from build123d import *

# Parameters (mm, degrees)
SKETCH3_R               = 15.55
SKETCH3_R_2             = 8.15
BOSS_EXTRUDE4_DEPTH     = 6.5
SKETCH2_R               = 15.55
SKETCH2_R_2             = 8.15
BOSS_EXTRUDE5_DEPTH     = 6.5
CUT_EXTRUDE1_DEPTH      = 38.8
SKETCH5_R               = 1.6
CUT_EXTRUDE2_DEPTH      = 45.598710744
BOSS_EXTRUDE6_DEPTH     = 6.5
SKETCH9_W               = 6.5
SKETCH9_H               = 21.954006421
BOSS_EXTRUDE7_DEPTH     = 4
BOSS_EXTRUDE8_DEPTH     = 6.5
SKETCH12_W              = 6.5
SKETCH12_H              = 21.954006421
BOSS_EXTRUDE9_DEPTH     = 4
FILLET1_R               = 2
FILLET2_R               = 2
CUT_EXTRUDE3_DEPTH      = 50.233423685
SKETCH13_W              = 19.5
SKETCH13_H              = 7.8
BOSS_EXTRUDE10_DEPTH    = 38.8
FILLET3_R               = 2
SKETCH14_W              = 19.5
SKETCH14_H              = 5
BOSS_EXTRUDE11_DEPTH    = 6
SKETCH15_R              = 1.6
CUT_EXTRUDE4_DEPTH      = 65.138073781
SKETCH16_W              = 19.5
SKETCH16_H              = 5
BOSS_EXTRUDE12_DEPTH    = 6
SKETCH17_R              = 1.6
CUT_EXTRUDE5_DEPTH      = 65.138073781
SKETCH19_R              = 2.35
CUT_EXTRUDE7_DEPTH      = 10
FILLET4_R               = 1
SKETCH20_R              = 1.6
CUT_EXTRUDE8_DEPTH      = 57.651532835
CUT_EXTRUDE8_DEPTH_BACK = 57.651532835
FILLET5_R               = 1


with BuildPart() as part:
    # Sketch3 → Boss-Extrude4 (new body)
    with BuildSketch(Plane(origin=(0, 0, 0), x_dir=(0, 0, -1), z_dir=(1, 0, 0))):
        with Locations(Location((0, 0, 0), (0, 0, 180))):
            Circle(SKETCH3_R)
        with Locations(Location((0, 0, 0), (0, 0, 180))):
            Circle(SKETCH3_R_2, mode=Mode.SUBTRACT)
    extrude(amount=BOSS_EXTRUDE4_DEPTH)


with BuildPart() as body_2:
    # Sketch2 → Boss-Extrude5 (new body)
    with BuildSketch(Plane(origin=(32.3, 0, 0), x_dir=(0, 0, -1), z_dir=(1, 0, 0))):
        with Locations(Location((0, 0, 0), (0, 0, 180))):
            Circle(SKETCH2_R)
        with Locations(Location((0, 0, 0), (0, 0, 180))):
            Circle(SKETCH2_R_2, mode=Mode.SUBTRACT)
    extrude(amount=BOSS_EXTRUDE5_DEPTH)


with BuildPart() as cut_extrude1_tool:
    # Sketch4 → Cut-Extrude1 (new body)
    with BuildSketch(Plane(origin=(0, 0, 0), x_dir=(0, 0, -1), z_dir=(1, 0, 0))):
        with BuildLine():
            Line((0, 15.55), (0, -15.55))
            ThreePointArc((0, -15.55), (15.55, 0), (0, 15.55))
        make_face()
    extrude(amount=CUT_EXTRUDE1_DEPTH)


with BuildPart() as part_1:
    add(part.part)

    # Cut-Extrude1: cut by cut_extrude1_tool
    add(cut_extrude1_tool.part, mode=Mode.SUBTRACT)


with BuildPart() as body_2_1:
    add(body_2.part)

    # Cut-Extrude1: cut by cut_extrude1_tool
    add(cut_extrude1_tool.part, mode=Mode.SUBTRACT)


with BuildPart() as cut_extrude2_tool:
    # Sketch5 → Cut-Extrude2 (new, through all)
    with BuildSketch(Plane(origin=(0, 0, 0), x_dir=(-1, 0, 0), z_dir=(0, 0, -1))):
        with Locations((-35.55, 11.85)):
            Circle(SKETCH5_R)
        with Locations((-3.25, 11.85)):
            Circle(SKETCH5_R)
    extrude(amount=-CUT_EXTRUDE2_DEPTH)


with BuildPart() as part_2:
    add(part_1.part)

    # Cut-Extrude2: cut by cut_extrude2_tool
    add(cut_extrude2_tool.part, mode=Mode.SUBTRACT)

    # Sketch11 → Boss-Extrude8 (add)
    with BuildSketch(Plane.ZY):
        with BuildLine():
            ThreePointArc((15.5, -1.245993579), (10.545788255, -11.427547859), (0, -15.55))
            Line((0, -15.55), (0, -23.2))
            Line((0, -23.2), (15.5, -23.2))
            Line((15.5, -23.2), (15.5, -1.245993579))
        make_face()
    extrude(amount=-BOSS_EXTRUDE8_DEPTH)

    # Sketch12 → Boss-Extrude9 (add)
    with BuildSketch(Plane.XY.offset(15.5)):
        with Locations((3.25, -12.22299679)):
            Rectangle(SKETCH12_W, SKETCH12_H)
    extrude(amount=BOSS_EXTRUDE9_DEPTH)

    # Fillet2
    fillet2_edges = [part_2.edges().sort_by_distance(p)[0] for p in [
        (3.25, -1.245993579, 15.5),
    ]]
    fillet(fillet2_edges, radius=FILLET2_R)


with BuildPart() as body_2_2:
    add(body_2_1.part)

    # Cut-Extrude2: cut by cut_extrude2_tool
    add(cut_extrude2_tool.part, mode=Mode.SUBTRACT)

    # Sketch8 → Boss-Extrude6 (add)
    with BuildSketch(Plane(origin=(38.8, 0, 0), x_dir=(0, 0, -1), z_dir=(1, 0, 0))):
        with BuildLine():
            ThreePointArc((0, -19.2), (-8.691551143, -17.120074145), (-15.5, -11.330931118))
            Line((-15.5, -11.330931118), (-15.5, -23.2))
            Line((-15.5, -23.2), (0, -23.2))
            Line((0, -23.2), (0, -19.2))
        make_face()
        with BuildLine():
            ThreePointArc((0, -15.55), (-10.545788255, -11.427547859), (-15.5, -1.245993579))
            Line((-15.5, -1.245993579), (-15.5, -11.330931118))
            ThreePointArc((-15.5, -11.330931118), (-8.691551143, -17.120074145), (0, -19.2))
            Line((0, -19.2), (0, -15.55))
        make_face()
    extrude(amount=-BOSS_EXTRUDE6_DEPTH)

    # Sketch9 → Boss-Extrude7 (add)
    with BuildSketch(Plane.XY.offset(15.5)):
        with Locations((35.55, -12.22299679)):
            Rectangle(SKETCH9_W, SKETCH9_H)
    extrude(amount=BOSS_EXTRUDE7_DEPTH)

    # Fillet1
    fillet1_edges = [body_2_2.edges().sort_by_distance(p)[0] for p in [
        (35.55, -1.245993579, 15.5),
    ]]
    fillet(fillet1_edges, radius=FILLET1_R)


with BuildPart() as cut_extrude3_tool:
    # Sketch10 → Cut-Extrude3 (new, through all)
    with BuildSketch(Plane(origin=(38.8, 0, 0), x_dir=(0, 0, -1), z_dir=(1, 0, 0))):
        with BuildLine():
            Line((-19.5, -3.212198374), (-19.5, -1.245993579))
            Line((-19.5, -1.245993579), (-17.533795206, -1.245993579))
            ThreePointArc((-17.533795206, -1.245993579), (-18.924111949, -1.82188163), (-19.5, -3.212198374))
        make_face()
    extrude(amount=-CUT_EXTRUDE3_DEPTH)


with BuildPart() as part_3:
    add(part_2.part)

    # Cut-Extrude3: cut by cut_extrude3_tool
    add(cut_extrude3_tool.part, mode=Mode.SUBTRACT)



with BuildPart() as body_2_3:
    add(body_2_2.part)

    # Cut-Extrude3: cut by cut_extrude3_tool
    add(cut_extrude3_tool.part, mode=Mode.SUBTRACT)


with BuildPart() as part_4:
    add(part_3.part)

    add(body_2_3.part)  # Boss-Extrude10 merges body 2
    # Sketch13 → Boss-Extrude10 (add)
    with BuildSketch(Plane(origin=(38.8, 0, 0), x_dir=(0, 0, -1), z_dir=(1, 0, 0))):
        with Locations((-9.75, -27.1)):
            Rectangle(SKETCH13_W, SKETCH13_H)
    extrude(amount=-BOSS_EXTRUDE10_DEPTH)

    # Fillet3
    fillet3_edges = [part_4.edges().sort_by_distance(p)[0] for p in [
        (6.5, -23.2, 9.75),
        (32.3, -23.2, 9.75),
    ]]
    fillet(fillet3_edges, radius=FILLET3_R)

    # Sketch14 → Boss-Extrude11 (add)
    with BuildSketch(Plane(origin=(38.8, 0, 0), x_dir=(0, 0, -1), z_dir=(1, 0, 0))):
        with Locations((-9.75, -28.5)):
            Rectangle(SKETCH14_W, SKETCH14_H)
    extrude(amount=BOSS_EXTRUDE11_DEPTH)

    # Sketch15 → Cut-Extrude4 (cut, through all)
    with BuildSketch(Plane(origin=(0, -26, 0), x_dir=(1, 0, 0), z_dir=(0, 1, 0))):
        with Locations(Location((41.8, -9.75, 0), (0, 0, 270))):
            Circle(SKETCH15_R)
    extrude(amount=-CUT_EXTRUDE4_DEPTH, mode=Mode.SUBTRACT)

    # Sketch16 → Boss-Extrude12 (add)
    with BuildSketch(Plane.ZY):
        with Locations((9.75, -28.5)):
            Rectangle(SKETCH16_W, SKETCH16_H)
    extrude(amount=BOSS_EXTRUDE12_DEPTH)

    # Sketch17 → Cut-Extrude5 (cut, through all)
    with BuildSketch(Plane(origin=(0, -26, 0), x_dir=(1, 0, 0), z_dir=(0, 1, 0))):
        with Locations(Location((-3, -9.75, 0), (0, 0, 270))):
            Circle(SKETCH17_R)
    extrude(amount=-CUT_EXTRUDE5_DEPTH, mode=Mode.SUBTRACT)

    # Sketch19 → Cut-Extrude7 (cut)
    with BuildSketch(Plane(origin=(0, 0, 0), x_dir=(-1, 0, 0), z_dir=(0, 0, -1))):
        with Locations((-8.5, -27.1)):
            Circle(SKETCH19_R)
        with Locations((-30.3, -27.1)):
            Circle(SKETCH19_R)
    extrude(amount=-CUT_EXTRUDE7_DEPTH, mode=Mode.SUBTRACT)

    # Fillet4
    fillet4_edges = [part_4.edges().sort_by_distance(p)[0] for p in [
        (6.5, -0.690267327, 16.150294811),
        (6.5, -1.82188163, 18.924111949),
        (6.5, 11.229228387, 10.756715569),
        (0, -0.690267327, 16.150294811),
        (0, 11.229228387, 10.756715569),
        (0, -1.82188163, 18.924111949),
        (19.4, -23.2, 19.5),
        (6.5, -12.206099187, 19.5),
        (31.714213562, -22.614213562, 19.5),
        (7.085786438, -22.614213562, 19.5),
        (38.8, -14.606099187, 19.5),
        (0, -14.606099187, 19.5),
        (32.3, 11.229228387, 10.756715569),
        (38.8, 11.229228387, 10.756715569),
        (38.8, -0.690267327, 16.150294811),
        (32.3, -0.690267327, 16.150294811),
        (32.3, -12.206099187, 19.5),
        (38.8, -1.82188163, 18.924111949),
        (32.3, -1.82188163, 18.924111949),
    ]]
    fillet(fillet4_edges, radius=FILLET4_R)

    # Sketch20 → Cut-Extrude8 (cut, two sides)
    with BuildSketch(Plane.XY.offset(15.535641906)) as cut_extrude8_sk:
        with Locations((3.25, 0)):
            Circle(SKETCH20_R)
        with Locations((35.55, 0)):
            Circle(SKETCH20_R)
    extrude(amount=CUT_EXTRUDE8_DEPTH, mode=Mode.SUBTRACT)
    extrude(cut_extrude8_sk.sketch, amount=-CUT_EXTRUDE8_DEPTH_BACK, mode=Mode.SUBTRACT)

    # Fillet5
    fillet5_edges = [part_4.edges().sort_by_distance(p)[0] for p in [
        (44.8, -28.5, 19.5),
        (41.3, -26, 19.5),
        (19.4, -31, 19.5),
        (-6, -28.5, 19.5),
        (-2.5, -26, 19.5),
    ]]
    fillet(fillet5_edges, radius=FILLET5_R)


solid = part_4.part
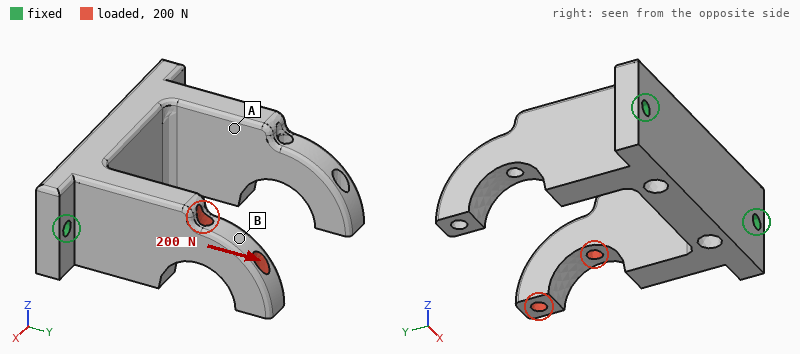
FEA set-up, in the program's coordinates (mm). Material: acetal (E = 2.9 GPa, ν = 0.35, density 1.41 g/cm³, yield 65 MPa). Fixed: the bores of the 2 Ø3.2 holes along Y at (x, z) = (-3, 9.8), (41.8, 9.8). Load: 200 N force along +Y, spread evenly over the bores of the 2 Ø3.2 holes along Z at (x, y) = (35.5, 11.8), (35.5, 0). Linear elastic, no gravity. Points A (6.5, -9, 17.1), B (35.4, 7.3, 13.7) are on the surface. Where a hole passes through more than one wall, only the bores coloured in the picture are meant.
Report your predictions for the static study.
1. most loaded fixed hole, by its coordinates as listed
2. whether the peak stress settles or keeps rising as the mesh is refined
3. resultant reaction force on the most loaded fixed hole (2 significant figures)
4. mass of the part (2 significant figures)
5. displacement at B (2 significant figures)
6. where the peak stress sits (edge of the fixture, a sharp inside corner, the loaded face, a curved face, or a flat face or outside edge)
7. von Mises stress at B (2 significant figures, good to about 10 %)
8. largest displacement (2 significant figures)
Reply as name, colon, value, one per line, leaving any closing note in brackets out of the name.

most loaded fixed hole, by its coordinates as listed: (41.8, 9.8)
whether the peak stress settles or keeps rising as the mesh is refined: keeps rising
resultant reaction force on the most loaded fixed hole: 180 N
mass of the part: 19 g
displacement at B: 0.19 mm
where the peak stress sits: a sharp inside corner
von Mises stress at B: 6.3 MPa
largest displacement: 0.49 mm
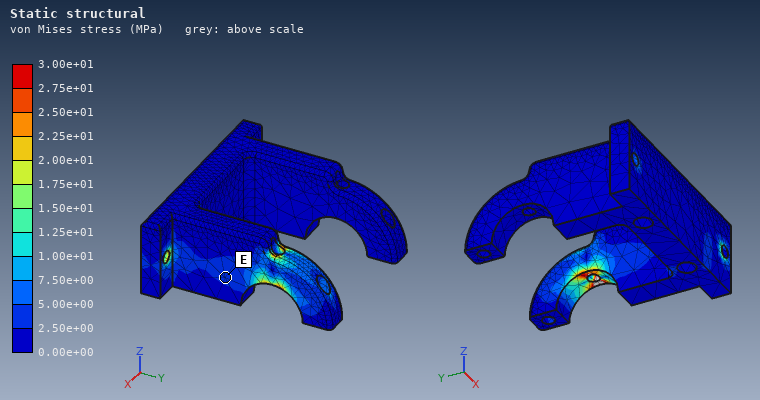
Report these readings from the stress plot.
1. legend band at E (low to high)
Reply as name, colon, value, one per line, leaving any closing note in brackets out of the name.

legend band at E: 2.50e+00 to 5.00e+00 MPa
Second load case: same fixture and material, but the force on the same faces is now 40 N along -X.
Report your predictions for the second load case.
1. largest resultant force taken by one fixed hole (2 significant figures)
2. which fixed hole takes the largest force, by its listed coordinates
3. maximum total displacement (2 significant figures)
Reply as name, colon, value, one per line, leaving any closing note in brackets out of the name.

largest resultant force taken by one fixed hole: 62 N
which fixed hole takes the largest force, by its listed coordinates: (-3, 9.8)
maximum total displacement: 0.81 mm
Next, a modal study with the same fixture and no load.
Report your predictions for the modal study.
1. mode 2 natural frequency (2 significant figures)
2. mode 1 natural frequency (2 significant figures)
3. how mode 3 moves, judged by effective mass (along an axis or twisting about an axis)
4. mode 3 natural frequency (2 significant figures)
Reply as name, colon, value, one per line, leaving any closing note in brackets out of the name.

mode 2 natural frequency: 1000 Hz
mode 1 natural frequency: 1000 Hz
how mode 3 moves, judged by effective mass: along X
mode 3 natural frequency: 1200 Hz
